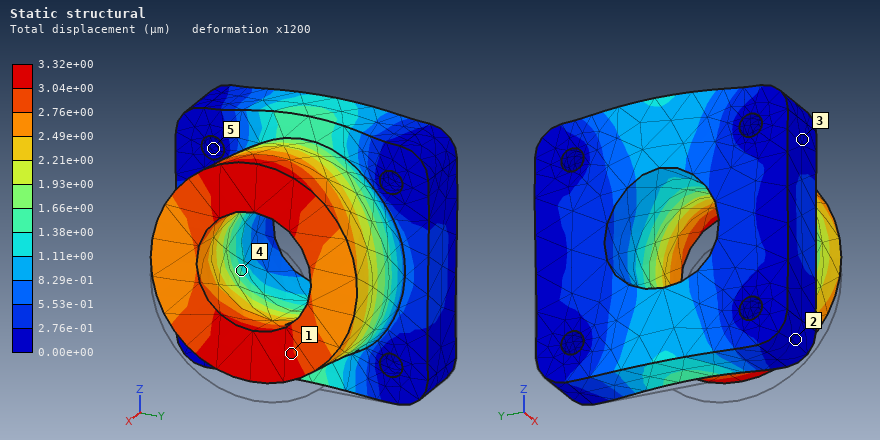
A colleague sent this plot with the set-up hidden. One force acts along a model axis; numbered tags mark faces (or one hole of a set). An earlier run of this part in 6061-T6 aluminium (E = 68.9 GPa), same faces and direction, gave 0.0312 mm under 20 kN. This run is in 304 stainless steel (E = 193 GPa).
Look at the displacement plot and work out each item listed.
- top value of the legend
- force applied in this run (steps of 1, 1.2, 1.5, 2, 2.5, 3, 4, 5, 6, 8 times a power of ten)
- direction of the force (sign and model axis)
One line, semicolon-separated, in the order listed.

3.32e+00 µm; 6 kN; +Z
